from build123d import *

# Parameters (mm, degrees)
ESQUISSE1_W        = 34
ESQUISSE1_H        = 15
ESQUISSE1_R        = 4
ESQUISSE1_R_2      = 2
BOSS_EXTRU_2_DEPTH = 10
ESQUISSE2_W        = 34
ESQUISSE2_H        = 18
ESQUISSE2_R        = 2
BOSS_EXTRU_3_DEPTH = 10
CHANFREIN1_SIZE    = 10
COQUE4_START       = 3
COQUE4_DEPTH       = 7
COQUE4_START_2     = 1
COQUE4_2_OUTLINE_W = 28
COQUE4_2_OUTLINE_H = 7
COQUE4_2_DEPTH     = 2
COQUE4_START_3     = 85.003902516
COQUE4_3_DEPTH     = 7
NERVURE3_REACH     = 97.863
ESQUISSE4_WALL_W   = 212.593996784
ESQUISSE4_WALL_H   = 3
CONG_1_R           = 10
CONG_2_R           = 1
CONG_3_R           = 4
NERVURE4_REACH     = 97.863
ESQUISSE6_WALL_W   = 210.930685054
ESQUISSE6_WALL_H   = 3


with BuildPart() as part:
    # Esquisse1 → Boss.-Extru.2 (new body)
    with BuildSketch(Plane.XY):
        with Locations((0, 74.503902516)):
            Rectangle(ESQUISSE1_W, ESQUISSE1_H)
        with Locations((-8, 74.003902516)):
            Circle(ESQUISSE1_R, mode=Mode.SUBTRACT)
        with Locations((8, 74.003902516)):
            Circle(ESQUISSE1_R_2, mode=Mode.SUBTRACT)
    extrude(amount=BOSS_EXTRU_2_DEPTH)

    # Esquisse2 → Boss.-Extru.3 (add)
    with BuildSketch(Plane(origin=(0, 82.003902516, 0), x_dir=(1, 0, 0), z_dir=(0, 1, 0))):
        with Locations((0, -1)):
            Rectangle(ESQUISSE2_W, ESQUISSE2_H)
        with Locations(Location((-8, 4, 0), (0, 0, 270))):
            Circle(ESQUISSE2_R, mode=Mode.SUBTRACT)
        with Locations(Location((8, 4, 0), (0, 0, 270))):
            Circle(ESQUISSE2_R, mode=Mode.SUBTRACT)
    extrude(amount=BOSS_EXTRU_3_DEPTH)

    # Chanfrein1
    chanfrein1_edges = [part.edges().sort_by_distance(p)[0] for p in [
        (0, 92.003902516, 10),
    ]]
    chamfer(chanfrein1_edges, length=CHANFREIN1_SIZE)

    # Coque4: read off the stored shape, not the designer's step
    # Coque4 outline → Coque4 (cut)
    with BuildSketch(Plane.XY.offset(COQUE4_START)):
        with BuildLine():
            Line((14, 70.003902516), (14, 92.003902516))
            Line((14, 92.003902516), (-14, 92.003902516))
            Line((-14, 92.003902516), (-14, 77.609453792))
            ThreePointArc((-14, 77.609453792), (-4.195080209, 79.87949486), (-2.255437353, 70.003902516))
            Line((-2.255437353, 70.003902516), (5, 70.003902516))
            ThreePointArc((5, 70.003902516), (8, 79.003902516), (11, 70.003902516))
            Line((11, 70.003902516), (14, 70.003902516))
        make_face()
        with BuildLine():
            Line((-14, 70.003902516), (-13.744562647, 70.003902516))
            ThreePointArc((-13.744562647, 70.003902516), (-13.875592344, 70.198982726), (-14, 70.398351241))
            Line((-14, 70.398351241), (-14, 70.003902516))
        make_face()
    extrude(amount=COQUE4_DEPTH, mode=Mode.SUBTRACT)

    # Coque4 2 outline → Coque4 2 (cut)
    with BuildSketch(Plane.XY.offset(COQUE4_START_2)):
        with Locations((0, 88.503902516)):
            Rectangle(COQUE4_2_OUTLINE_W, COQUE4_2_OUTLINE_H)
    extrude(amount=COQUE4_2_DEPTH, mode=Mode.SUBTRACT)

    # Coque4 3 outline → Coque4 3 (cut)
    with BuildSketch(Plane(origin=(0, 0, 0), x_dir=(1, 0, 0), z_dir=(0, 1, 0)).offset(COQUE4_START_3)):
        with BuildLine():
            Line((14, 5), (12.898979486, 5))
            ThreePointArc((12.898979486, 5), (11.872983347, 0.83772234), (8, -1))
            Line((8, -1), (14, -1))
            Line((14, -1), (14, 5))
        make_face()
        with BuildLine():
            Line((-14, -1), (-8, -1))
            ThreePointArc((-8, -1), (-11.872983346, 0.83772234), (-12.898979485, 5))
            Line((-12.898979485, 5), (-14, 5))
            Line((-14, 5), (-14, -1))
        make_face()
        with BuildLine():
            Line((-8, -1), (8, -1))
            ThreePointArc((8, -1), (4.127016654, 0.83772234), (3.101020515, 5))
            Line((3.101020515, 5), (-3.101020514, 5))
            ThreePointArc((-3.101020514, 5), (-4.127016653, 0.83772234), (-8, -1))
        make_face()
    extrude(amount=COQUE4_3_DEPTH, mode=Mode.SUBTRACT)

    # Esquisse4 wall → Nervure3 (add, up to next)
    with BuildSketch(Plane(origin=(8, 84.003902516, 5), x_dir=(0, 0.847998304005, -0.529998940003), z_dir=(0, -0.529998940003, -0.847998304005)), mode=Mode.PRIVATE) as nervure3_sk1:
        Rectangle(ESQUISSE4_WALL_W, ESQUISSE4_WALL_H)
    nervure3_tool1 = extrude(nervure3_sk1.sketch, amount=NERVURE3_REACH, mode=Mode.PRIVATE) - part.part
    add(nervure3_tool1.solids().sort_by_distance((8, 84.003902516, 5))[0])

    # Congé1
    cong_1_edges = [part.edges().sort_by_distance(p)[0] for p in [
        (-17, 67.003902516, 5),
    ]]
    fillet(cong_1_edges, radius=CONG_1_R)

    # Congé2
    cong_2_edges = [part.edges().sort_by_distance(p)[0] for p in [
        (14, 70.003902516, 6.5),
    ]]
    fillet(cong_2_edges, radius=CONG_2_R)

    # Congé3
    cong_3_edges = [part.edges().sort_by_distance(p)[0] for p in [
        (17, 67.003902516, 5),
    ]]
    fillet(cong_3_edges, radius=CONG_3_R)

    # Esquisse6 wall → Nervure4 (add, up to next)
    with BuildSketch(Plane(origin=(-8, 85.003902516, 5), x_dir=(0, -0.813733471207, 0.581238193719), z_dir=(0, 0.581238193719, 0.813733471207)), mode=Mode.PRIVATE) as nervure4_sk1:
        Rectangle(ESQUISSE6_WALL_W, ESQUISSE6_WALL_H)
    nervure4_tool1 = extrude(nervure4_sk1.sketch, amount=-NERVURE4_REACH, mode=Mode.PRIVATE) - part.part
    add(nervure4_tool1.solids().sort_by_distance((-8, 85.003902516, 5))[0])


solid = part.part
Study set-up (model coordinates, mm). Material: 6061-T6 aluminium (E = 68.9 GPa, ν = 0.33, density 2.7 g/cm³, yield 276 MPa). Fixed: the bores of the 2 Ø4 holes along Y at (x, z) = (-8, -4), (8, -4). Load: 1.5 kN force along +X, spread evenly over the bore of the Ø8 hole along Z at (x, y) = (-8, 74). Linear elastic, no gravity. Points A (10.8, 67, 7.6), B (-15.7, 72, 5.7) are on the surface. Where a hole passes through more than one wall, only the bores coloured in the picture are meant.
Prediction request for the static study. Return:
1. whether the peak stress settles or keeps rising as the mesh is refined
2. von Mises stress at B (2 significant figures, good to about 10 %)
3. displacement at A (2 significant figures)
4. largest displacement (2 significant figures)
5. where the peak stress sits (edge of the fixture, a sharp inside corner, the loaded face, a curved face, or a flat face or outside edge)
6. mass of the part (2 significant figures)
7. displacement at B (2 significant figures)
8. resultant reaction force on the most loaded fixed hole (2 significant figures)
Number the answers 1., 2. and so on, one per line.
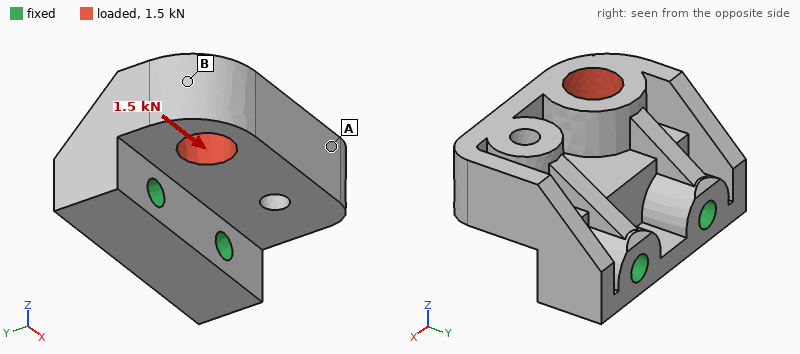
1. keeps rising
2. 9.1 MPa
3. 18 µm
4. 23 µm
5. edge of the fixture
6. 17 g
7. 20 µm
8. 1.2 kN
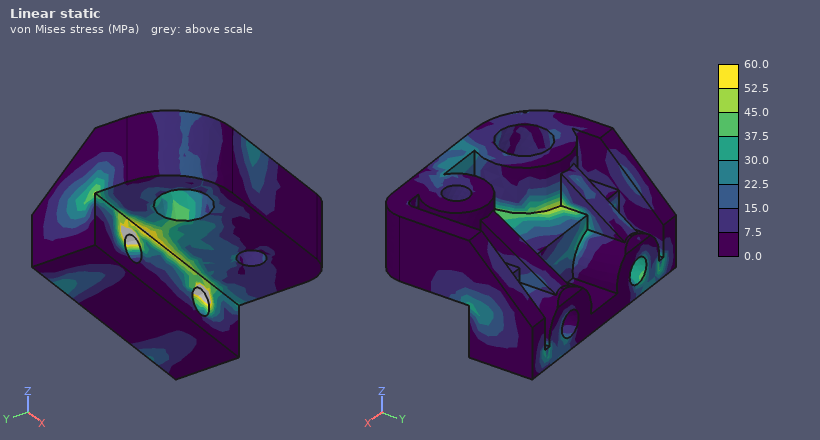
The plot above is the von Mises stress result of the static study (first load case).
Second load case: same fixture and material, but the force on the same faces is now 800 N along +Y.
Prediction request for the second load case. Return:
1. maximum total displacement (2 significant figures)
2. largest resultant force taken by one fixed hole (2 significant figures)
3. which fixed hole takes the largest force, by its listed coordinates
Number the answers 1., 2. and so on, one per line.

1. 32 µm
2. 720 N
3. (-8, -4)
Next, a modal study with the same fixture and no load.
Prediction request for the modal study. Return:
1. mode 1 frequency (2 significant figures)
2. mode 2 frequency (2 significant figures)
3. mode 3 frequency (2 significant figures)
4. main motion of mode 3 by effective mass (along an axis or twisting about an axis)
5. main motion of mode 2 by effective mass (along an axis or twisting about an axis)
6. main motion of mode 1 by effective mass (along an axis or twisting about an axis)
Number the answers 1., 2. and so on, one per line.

1. 7900 Hz
2. 13 kHz
3. 16 kHz
4. along X
5. twisting about Y
6. along Z
